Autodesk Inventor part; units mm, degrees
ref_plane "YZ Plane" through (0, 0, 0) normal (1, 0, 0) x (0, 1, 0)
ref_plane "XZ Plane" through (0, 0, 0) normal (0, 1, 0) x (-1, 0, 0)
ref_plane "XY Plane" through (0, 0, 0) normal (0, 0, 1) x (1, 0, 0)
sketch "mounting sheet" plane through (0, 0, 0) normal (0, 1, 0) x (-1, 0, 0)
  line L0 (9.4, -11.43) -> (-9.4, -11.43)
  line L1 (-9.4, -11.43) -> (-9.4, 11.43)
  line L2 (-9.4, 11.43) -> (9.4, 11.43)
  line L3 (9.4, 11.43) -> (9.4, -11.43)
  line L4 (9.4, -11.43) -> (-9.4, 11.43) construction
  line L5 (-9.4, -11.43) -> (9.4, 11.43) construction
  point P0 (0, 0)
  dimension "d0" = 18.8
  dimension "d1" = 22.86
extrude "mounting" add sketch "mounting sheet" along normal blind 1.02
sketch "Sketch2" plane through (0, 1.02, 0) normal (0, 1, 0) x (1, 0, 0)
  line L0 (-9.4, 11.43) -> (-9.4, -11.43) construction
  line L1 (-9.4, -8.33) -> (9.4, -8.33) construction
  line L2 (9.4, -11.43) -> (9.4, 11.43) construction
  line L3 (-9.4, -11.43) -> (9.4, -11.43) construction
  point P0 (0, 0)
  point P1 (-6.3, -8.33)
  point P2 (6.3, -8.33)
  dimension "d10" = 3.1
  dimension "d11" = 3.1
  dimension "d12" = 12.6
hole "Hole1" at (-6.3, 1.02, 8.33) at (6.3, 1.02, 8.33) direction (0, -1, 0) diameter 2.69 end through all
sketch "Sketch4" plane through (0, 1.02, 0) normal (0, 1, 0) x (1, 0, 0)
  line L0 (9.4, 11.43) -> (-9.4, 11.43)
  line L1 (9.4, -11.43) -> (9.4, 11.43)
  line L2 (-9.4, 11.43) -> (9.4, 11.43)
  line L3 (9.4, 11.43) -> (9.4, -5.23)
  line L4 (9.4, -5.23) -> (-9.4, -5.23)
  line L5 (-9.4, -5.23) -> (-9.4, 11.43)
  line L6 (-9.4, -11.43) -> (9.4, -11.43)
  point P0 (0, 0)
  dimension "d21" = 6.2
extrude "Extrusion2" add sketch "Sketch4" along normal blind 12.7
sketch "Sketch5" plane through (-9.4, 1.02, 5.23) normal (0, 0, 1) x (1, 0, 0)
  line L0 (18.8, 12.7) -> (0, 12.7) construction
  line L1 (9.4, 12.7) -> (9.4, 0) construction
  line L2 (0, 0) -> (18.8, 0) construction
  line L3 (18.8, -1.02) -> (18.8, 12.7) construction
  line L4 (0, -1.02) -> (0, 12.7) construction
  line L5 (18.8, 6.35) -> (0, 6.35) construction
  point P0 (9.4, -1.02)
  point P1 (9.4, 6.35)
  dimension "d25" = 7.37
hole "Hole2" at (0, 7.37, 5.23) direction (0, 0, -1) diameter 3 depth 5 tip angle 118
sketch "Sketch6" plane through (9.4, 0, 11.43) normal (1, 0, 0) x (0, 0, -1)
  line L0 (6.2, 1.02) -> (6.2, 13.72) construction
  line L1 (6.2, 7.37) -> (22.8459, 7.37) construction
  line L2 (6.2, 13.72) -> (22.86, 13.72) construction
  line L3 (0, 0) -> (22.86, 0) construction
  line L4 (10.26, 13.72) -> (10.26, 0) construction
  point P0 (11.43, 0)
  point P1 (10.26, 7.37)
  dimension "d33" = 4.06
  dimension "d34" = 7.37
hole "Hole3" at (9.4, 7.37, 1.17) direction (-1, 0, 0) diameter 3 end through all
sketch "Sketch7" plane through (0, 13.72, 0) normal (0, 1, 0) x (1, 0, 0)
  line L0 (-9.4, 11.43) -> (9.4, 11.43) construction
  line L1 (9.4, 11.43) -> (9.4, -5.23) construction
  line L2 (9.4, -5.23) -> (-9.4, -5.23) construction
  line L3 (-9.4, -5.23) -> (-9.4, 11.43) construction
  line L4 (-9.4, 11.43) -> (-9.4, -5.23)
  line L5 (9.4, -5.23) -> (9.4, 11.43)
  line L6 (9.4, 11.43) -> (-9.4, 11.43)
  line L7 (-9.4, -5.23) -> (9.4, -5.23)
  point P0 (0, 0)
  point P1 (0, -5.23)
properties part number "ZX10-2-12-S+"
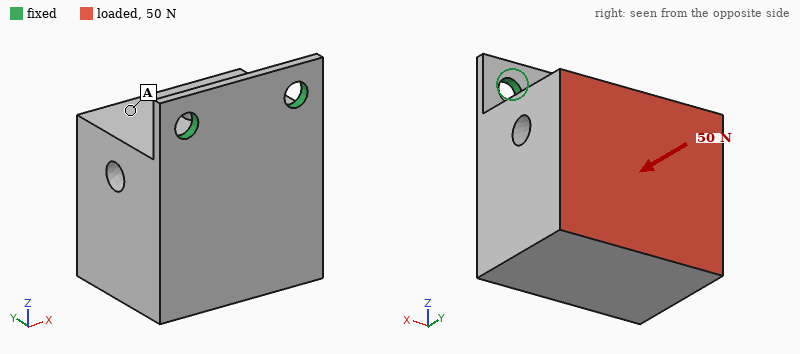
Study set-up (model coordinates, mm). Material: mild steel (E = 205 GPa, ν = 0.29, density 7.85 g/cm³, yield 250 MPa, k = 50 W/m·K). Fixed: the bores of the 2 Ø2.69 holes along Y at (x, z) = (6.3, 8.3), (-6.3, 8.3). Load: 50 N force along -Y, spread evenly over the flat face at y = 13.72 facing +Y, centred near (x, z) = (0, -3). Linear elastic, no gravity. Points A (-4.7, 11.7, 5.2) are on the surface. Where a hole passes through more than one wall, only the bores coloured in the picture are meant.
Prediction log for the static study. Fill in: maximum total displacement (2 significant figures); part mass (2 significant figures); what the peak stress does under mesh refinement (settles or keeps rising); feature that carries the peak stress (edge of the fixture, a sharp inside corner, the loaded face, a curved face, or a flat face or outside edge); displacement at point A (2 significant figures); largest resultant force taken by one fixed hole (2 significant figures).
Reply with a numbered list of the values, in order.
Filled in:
1. 85 µm
2. 33 g
3. keeps rising
4. edge of the fixture
5. 43 µm
6. 25 N
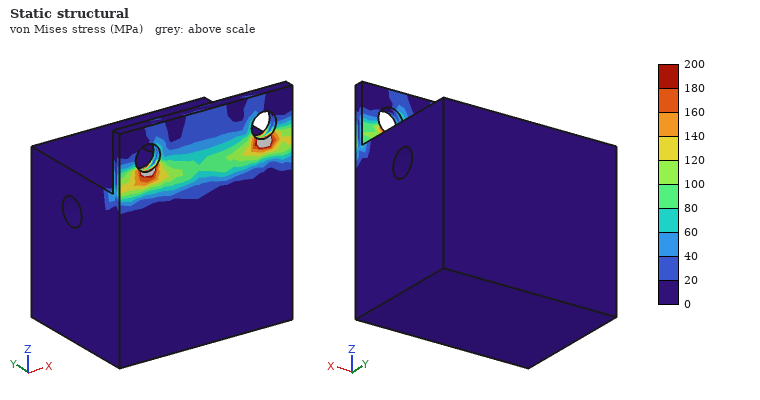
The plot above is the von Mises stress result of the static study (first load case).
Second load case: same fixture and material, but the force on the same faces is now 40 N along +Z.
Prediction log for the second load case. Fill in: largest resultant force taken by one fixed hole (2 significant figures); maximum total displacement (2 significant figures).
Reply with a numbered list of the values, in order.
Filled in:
1. 20 N
2. 96 µm
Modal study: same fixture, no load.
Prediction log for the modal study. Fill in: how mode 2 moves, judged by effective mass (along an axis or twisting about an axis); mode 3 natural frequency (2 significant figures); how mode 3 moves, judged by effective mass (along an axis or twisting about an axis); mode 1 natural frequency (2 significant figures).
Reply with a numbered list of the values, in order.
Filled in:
1. along X
2. 11 kHz
3. along X
4. 750 Hz
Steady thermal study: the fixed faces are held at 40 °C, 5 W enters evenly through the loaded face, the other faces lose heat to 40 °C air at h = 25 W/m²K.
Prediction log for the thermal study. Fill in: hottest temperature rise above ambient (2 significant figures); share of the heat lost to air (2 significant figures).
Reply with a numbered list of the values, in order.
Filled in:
1. 26 K
2. 17 %
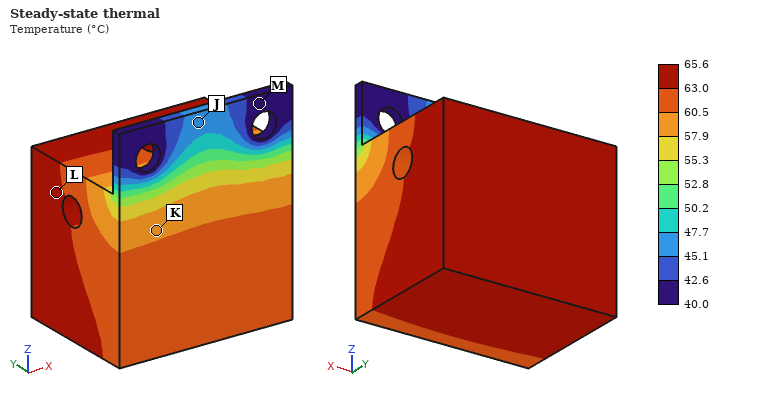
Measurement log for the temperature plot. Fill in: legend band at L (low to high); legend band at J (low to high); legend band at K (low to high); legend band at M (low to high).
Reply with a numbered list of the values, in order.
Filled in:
1. 63.0 to 65.6 °C
2. 45.1 to 47.7 °C
3. 57.9 to 60.5 °C
4. 40.0 to 42.6 °C
